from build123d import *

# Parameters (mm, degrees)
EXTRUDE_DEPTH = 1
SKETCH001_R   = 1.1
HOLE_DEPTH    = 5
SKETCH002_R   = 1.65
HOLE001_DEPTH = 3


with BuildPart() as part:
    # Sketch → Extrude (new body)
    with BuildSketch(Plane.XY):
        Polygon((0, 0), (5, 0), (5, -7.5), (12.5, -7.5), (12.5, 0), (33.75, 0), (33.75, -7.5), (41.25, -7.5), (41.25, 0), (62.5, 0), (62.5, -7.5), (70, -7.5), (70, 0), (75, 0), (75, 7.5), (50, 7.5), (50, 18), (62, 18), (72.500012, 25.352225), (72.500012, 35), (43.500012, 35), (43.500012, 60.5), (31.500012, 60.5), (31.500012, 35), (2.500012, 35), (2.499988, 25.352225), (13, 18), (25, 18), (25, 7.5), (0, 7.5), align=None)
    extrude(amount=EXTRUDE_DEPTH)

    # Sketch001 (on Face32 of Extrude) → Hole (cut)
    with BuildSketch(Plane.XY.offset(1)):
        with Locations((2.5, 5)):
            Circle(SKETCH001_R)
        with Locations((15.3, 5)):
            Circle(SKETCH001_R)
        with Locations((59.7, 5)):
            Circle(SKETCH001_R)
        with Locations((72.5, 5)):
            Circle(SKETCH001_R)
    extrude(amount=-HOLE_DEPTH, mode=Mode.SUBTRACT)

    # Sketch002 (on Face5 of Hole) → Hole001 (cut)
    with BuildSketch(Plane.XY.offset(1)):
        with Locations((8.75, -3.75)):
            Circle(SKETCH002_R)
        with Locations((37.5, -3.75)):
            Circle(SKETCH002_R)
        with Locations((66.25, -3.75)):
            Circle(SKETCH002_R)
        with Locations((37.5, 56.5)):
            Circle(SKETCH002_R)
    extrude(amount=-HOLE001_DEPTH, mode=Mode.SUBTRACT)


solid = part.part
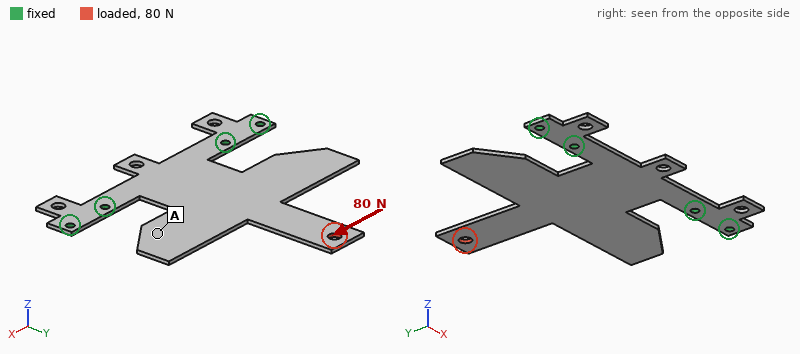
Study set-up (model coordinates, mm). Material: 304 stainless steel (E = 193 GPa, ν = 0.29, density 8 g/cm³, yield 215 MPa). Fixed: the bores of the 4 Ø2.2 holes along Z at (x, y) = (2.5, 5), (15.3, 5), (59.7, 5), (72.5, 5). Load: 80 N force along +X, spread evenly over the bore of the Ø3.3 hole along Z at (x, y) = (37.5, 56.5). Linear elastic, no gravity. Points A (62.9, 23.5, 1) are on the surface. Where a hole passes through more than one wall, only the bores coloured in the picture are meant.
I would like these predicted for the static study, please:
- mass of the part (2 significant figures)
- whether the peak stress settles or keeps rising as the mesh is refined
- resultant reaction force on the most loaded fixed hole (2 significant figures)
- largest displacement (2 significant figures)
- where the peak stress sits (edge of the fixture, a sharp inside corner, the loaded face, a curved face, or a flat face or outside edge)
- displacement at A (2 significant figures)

19 g
keeps rising
140 N
58 µm
a sharp inside corner
20 µm
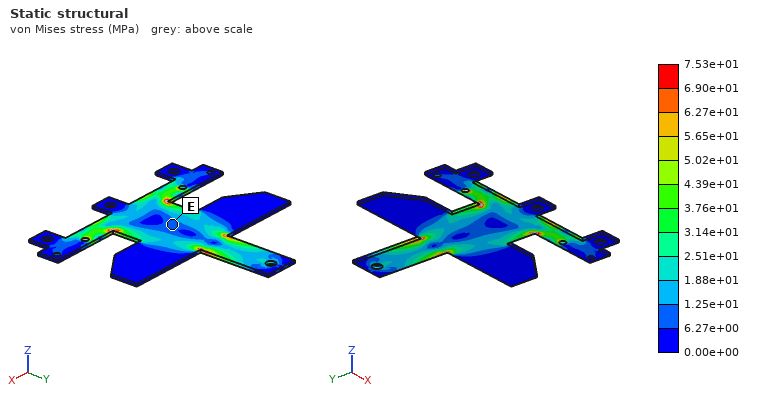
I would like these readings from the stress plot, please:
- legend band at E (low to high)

6.27e+00 to 1.25e+01 MPa
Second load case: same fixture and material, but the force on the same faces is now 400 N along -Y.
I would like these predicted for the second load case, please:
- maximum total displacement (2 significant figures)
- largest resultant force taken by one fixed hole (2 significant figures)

22 µm
250 N
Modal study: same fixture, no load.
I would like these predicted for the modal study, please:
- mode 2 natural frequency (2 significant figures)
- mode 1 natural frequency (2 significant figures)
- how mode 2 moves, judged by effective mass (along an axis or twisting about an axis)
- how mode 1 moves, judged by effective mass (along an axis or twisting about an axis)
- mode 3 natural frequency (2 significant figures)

520 Hz
210 Hz
twisting about Y
along Z
800 Hz
